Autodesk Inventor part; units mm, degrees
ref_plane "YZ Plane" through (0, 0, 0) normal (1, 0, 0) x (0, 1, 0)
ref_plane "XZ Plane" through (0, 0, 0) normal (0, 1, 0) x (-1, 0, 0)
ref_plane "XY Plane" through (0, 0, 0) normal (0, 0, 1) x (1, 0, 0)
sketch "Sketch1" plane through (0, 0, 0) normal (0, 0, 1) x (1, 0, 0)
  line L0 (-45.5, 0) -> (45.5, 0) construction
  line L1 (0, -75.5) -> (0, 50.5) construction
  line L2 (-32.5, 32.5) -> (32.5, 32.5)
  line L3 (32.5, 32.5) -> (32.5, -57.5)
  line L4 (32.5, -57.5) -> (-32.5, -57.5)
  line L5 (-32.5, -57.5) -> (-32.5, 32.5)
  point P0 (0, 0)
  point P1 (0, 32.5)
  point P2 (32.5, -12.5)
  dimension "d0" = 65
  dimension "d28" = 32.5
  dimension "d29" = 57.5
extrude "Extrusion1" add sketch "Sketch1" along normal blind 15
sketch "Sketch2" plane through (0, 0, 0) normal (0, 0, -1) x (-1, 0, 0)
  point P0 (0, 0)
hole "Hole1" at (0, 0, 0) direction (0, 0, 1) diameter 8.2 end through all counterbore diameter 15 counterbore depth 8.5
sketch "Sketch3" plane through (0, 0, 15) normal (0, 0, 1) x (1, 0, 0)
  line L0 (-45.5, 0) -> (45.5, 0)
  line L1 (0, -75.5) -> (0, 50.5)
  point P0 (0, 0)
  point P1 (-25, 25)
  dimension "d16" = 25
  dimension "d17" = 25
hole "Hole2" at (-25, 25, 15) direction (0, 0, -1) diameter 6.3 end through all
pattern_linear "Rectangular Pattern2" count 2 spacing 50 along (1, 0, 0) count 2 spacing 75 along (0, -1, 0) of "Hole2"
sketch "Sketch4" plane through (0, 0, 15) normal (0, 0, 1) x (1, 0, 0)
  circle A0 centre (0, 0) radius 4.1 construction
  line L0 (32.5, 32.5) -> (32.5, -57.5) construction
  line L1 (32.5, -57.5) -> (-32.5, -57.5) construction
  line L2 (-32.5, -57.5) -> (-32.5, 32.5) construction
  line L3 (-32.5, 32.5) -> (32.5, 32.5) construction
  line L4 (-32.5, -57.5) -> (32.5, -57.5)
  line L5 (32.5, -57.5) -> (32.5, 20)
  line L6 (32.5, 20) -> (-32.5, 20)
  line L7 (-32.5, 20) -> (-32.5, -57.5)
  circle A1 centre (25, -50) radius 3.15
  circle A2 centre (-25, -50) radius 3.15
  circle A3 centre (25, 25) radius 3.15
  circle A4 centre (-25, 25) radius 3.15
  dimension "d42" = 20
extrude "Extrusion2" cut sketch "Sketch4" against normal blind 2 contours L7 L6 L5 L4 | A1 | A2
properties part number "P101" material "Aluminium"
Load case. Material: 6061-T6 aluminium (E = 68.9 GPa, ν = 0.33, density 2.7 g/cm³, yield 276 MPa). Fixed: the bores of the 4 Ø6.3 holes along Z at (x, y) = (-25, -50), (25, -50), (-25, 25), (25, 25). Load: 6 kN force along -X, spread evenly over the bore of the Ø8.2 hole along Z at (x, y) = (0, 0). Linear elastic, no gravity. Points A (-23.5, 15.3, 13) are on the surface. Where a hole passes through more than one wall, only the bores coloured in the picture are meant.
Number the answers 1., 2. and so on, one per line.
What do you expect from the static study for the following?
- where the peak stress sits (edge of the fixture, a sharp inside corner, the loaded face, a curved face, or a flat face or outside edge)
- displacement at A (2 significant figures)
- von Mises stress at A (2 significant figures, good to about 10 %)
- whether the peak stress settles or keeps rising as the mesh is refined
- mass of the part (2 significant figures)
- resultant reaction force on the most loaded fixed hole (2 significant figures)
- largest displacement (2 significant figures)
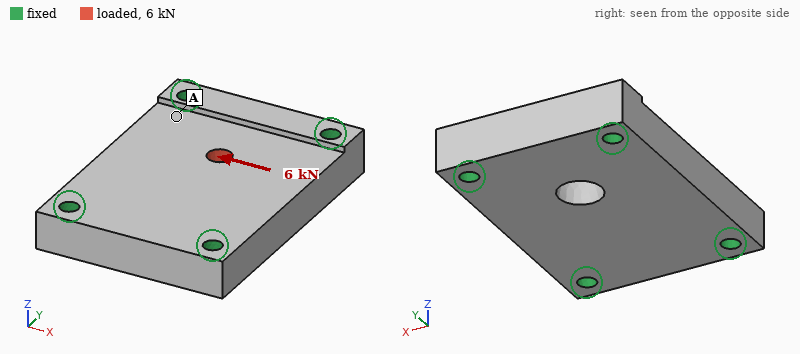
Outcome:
1. a sharp inside corner
2. 2.4 µm
3. 11 MPa
4. keeps rising
5. 200 g
6. 2.3 kN
7. 12 µm
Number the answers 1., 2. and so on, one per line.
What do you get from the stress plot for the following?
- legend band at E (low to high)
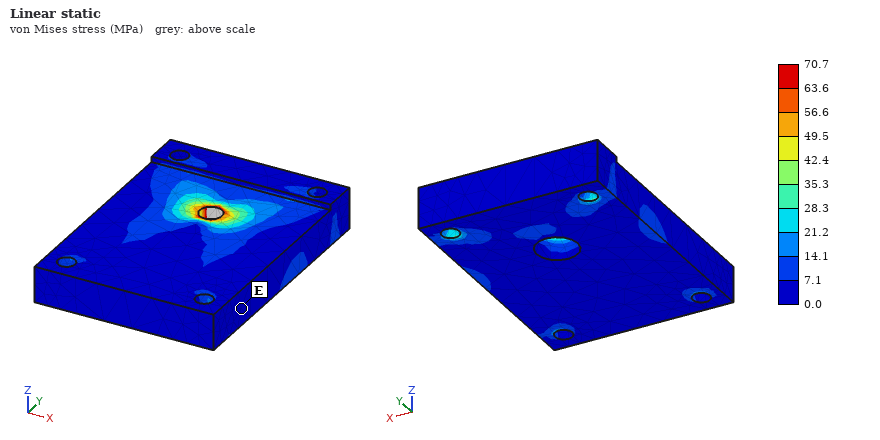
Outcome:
1. 0.0 to 7.1 MPa
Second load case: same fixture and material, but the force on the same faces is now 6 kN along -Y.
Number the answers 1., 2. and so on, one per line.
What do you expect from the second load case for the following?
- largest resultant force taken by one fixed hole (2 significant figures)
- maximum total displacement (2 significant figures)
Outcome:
1. 2.0 kN
2. 11 µm
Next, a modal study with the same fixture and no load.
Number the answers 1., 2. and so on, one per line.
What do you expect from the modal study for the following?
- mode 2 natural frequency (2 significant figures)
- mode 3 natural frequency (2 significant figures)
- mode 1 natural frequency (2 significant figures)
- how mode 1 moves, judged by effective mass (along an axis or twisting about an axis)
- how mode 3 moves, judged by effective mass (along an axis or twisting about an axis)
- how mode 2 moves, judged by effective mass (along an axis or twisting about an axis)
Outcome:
1. 12 kHz
2. 17 kHz
3. 9000 Hz
4. along Z
5. along X
6. twisting about Y
